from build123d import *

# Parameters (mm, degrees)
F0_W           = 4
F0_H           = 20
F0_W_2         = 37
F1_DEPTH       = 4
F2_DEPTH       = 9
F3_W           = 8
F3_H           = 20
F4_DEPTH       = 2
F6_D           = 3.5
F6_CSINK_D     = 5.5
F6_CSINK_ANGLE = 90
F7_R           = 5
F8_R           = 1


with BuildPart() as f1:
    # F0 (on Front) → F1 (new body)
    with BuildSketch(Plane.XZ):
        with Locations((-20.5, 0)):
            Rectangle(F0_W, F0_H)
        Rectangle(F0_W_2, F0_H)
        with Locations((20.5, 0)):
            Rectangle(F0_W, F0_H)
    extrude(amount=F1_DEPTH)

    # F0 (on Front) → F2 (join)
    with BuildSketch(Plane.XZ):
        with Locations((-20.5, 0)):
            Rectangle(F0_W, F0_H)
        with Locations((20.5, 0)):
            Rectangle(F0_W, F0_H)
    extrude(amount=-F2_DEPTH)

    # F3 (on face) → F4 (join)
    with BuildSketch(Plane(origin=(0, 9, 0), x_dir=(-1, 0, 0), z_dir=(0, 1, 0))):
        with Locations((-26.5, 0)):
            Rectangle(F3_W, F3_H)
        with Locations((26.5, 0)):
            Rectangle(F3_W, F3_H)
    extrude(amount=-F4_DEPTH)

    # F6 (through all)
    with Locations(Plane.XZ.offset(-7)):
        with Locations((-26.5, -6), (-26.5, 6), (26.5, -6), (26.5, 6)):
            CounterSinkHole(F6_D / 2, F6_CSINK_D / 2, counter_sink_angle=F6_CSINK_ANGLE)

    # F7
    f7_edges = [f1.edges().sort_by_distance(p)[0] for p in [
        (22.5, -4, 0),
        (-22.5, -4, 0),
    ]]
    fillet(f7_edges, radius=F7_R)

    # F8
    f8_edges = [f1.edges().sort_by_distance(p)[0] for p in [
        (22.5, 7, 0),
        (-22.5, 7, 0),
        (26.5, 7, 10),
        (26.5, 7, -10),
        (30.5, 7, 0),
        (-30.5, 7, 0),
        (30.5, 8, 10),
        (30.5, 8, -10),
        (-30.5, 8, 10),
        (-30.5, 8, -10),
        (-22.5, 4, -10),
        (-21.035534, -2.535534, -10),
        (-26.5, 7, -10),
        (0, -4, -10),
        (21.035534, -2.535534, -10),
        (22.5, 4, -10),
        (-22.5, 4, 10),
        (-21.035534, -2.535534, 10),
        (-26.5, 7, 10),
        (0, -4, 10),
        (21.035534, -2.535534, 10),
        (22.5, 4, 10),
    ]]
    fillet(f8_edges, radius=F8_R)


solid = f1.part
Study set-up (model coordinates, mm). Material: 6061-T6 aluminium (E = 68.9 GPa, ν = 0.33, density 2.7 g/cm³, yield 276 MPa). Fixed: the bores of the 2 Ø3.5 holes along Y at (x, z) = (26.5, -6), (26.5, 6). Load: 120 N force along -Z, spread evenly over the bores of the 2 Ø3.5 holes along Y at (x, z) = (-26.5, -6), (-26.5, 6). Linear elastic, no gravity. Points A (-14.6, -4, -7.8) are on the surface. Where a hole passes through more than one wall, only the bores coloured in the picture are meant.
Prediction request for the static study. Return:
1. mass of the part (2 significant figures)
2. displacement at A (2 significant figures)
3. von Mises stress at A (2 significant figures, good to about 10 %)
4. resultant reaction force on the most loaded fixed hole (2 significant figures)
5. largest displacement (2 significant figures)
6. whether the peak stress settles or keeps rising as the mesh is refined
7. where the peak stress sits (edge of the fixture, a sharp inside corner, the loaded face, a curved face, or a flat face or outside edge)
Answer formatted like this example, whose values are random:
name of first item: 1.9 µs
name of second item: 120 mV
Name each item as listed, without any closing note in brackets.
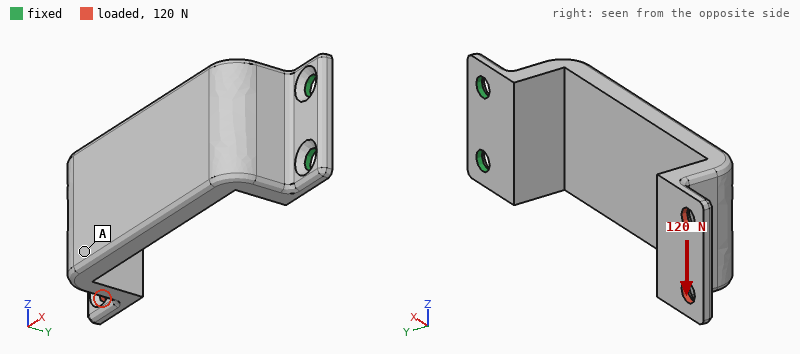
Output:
mass of the part: 14 g
displacement at A: 0.18 mm
von Mises stress at A: 14 MPa
resultant reaction force on the most loaded fixed hole: 450 N
largest displacement: 0.38 mm
whether the peak stress settles or keeps rising as the mesh is refined: keeps rising
where the peak stress sits: edge of the fixture
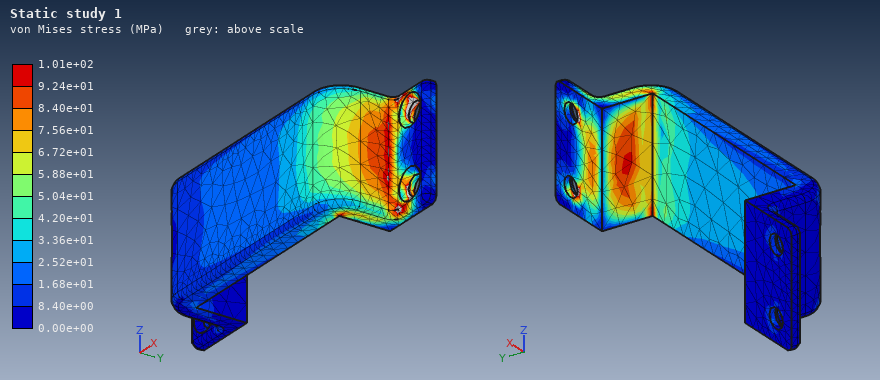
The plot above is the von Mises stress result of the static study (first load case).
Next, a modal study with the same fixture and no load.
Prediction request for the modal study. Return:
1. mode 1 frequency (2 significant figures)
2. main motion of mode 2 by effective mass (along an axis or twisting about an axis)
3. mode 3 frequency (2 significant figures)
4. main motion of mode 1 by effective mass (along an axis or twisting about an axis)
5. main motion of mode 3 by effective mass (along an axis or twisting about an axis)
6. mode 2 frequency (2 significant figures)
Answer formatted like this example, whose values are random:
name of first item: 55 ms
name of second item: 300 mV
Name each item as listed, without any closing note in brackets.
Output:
mode 1 frequency: 500 Hz
main motion of mode 2 by effective mass: along Z
mode 3 frequency: 3100 Hz
main motion of mode 1 by effective mass: along Y
main motion of mode 3 by effective mass: along X
mode 2 frequency: 1600 Hz
